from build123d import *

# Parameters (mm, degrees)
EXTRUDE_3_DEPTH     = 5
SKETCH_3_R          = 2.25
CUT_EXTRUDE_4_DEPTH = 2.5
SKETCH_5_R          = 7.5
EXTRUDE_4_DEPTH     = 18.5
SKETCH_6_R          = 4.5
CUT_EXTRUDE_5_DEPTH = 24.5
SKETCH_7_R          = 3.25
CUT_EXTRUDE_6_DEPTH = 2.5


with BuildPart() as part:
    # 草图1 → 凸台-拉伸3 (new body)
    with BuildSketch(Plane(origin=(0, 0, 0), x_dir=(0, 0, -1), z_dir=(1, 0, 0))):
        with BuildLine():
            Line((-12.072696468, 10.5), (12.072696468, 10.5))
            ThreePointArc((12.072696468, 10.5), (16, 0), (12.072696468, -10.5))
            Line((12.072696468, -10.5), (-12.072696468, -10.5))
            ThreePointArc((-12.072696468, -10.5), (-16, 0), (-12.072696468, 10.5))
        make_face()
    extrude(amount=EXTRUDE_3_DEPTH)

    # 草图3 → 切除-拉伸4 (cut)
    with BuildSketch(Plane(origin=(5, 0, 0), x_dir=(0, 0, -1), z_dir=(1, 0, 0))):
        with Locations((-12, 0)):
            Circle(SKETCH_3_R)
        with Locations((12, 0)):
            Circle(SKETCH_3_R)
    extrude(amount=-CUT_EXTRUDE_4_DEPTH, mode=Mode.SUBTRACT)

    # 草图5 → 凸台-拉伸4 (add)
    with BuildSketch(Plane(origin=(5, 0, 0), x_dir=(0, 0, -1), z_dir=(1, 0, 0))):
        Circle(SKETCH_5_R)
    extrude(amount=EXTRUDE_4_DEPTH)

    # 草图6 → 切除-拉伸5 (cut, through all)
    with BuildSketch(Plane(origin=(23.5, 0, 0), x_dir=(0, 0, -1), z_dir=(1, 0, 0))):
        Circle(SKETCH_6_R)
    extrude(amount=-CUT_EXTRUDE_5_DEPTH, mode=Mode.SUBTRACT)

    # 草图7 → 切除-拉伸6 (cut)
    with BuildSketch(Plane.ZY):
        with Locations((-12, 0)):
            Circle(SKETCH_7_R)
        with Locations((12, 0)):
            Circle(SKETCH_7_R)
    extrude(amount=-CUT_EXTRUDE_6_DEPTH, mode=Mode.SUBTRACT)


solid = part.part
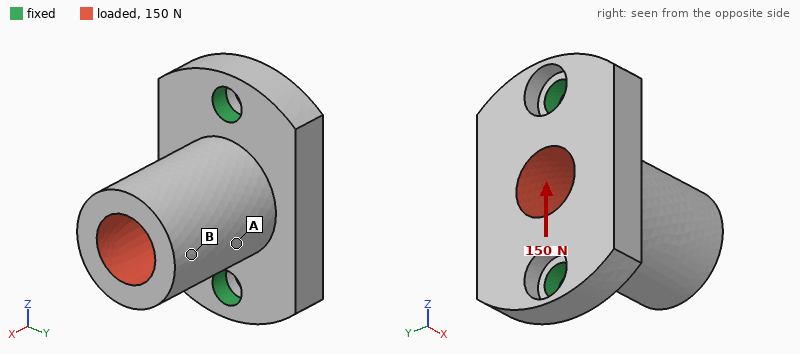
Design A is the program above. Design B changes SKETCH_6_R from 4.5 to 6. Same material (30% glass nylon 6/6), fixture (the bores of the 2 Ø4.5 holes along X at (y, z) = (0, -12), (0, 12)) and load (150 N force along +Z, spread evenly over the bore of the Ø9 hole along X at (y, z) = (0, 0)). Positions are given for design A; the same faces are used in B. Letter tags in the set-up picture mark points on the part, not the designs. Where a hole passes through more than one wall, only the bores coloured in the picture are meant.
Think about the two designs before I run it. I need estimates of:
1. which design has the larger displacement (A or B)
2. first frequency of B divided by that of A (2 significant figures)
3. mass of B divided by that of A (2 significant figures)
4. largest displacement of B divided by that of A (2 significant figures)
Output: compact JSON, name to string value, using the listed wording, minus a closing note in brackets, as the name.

{"which design has the larger displacement": "B", "first frequency of B divided by that of A": "1.2", "mass of B divided by that of A": "0.75", "largest displacement of B divided by that of A": "1.5"}
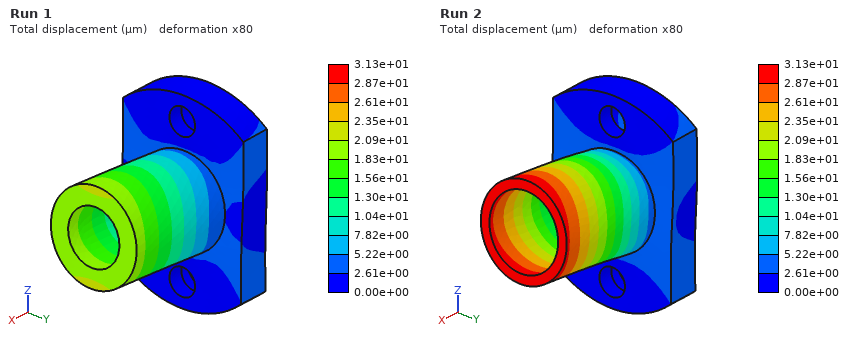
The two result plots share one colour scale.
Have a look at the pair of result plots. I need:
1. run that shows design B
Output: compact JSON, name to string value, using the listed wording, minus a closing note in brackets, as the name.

{"run that shows design B": "Run 2"}
